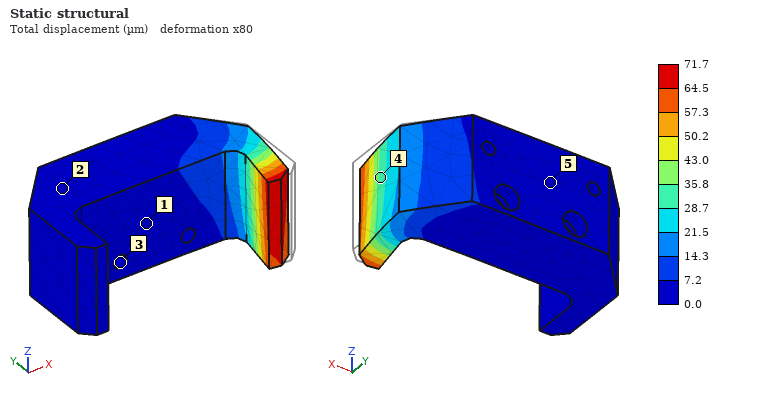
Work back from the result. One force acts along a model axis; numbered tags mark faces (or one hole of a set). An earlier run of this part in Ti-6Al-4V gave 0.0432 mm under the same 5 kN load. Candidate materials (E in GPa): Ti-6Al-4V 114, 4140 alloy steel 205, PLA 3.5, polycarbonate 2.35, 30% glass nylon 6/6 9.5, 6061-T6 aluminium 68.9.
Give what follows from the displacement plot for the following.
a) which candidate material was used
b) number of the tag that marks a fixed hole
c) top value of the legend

6061-T6 aluminium
3
71.7 µm
